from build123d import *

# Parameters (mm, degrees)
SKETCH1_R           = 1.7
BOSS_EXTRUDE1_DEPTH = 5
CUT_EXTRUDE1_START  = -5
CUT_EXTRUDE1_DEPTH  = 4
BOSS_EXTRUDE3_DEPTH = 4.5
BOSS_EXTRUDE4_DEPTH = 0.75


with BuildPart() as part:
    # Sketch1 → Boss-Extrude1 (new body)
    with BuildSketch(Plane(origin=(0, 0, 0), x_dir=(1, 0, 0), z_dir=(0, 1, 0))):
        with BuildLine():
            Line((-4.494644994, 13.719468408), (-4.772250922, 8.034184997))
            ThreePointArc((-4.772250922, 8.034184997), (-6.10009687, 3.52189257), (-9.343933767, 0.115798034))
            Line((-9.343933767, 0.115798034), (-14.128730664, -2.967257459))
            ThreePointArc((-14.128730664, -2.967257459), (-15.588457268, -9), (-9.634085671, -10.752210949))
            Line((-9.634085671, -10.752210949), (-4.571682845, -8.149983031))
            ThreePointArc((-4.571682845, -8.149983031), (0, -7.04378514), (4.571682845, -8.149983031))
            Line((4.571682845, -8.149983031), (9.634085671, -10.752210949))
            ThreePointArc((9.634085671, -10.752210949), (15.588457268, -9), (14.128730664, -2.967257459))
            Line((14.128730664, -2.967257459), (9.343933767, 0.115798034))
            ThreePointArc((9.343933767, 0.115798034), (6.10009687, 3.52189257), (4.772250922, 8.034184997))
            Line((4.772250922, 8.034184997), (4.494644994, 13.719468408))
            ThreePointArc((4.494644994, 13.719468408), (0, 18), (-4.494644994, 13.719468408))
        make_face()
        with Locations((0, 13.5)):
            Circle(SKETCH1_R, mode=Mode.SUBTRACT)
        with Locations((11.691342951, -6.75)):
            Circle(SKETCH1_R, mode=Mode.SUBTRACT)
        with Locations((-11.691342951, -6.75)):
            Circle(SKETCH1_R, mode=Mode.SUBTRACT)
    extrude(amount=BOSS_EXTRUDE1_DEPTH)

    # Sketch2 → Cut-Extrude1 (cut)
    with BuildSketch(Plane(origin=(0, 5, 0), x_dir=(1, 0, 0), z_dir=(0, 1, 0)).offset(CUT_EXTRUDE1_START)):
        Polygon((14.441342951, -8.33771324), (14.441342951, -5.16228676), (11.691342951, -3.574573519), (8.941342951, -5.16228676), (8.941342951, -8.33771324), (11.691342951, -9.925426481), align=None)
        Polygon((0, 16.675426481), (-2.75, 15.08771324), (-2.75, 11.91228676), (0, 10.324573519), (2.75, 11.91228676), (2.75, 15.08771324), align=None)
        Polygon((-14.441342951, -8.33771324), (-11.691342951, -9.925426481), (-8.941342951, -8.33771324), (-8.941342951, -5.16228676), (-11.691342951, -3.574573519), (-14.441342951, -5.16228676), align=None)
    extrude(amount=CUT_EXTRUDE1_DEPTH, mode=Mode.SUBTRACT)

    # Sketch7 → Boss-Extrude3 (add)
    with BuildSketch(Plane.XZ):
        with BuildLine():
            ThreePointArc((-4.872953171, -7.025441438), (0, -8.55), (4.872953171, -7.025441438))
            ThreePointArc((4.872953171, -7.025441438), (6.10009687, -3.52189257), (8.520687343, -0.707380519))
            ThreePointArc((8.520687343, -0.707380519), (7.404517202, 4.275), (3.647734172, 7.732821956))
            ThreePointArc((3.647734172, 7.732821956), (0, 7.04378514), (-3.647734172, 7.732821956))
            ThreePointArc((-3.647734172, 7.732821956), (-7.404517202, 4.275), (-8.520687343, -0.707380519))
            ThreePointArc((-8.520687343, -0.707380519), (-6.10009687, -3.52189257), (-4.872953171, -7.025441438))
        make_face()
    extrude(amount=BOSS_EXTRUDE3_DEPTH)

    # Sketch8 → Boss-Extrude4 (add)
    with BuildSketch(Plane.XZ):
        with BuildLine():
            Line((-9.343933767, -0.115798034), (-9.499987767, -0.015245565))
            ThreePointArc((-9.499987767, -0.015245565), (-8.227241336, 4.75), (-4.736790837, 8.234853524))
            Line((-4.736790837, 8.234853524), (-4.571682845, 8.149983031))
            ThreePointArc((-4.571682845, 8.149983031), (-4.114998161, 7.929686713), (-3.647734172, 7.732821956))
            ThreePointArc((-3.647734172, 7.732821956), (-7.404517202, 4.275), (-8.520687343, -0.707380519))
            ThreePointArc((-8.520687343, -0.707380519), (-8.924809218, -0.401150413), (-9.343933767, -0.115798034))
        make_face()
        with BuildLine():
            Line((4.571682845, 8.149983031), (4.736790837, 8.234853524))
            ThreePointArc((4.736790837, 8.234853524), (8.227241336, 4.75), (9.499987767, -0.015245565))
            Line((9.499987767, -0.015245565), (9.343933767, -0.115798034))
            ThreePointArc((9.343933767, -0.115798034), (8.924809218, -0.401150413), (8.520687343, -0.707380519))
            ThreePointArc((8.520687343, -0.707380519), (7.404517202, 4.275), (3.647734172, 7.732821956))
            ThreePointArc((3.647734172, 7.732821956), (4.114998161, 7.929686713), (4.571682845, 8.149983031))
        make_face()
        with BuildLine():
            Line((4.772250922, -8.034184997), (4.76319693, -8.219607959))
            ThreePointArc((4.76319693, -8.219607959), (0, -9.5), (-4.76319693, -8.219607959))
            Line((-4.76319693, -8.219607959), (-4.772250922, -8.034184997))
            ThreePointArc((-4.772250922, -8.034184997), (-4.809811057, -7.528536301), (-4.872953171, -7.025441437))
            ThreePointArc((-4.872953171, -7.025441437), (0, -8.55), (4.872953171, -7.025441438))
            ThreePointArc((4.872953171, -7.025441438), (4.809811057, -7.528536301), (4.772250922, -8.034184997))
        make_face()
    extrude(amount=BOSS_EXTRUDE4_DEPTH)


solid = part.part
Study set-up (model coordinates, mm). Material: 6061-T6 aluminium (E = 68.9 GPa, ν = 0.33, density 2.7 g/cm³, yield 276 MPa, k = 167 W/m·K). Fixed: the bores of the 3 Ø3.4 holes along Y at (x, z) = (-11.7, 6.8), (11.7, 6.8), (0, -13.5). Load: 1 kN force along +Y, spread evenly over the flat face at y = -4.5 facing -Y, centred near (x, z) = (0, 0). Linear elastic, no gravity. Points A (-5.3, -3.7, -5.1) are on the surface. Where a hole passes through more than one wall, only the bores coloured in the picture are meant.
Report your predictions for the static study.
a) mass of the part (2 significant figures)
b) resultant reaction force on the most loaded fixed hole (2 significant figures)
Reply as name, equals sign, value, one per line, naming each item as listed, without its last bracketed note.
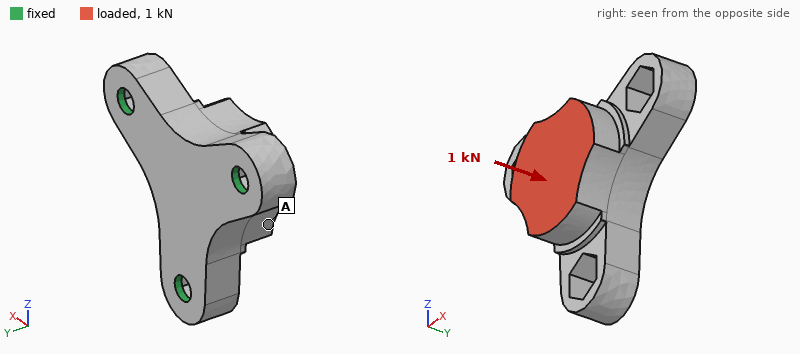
mass of the part = 7.8 g
resultant reaction force on the most loaded fixed hole = 420 N
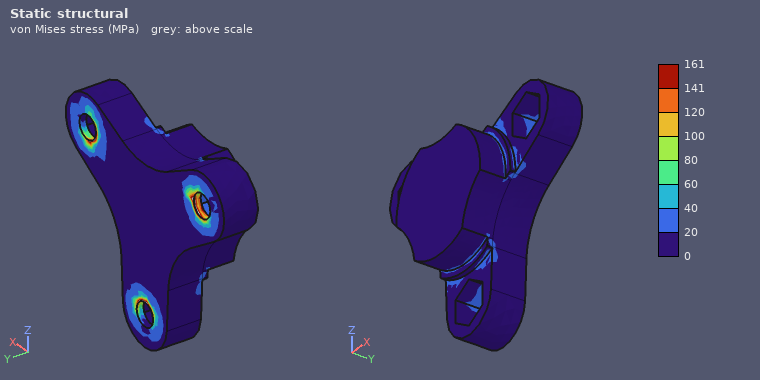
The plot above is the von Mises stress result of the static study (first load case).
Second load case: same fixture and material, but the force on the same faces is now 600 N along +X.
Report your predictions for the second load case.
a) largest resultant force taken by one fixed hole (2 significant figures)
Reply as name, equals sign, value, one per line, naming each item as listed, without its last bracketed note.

largest resultant force taken by one fixed hole = 380 N
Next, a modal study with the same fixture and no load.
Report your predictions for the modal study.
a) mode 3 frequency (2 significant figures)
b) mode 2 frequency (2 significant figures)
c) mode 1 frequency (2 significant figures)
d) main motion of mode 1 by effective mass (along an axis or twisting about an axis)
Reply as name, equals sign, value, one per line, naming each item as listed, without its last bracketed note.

mode 3 frequency = 29 kHz
mode 2 frequency = 29 kHz
mode 1 frequency = 23 kHz
main motion of mode 1 by effective mass = along Y
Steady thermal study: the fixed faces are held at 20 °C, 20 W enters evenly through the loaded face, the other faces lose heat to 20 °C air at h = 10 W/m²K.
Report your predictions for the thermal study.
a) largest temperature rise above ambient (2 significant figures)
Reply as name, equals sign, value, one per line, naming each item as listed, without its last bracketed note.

largest temperature rise above ambient = 15 K
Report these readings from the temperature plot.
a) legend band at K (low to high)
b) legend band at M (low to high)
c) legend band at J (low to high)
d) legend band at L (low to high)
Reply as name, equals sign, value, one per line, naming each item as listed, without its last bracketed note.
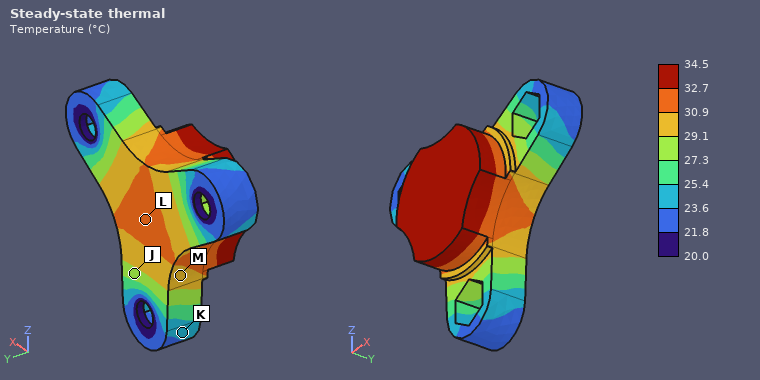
legend band at K = 23.6 to 25.4 °C
legend band at M = 29.1 to 30.9 °C
legend band at J = 27.3 to 29.1 °C
legend band at L = 30.9 to 32.7 °C
